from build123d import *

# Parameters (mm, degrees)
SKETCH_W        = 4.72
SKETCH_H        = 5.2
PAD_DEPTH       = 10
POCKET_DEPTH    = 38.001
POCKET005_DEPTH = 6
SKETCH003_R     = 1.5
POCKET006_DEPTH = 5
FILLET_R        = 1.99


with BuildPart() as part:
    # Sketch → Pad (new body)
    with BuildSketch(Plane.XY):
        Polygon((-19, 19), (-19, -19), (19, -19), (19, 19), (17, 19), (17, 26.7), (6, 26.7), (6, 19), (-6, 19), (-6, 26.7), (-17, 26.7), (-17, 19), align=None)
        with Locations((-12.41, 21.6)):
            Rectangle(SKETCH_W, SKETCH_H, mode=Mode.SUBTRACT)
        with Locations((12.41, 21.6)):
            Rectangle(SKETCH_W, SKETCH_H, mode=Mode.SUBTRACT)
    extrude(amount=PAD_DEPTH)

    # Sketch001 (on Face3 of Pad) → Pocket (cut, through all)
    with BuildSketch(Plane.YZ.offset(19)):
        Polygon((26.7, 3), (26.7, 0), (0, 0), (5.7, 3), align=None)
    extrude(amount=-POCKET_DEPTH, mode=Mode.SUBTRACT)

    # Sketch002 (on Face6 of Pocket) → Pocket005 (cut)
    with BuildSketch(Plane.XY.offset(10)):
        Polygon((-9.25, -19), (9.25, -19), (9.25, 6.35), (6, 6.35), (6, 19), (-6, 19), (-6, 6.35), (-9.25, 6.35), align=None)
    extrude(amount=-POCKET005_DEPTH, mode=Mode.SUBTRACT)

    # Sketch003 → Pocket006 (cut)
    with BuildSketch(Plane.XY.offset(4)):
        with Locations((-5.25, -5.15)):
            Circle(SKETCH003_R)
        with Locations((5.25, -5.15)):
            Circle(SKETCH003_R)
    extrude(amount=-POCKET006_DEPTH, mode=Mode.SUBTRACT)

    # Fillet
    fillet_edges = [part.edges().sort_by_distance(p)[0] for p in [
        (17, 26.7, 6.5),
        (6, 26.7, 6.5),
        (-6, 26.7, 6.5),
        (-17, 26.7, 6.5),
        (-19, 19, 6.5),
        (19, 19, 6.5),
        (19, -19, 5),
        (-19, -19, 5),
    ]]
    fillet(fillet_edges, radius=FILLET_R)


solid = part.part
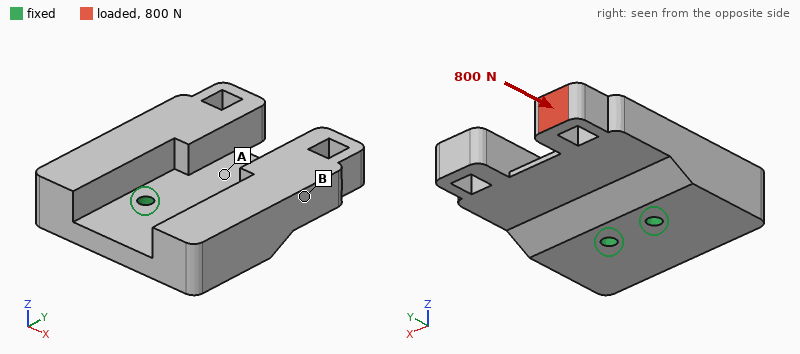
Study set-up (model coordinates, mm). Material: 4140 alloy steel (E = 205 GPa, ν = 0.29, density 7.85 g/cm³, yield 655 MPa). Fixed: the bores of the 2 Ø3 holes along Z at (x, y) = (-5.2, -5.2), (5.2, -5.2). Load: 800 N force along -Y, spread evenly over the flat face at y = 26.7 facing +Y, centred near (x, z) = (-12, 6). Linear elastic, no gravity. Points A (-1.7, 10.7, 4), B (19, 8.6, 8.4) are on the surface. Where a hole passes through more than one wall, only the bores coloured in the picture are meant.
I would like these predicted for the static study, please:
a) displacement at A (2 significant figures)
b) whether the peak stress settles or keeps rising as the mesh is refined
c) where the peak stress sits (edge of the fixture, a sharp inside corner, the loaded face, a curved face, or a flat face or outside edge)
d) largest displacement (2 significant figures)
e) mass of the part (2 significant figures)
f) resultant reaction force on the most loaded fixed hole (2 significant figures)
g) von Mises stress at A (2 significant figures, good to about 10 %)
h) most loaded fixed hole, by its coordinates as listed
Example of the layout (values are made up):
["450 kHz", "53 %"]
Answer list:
["6.7 µm", "keeps rising", "edge of the fixture", "22 µm", "75 g", "1.1 kN", "19 MPa", "(-5.2, -5.2)"]
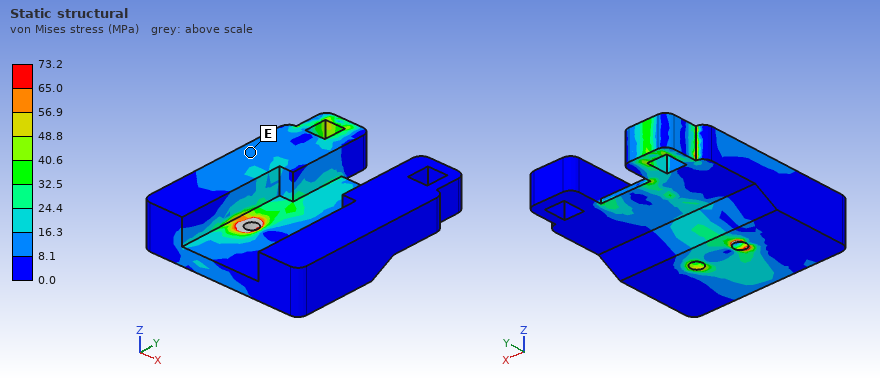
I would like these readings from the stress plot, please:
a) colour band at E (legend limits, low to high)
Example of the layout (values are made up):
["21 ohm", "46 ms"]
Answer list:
["8.1 to 16.3 MPa"]
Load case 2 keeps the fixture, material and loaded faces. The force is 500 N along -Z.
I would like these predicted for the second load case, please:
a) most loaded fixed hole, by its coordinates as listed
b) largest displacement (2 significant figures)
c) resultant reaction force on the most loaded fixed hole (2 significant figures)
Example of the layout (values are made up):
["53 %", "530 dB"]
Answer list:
["(-5.2, -5.2)", "0.13 mm", "600 N"]
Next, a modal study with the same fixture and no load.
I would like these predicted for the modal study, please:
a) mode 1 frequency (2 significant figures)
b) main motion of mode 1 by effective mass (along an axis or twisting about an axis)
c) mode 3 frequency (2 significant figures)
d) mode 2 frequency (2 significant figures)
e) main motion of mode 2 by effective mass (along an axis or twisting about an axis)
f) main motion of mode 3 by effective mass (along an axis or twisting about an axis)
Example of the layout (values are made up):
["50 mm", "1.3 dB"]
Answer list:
["3900 Hz", "along Z", "7000 Hz", "4600 Hz", "twisting about Y", "along X"]
